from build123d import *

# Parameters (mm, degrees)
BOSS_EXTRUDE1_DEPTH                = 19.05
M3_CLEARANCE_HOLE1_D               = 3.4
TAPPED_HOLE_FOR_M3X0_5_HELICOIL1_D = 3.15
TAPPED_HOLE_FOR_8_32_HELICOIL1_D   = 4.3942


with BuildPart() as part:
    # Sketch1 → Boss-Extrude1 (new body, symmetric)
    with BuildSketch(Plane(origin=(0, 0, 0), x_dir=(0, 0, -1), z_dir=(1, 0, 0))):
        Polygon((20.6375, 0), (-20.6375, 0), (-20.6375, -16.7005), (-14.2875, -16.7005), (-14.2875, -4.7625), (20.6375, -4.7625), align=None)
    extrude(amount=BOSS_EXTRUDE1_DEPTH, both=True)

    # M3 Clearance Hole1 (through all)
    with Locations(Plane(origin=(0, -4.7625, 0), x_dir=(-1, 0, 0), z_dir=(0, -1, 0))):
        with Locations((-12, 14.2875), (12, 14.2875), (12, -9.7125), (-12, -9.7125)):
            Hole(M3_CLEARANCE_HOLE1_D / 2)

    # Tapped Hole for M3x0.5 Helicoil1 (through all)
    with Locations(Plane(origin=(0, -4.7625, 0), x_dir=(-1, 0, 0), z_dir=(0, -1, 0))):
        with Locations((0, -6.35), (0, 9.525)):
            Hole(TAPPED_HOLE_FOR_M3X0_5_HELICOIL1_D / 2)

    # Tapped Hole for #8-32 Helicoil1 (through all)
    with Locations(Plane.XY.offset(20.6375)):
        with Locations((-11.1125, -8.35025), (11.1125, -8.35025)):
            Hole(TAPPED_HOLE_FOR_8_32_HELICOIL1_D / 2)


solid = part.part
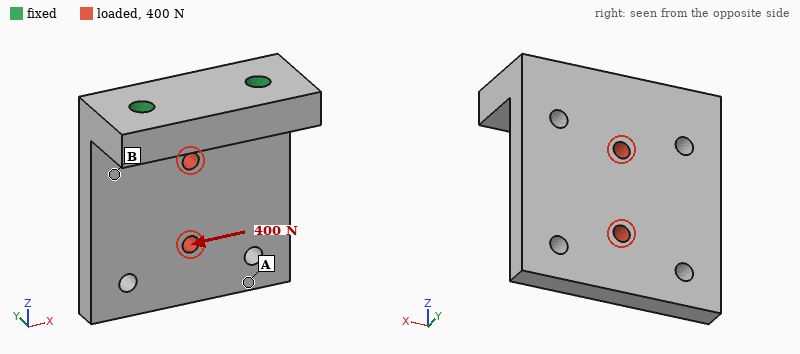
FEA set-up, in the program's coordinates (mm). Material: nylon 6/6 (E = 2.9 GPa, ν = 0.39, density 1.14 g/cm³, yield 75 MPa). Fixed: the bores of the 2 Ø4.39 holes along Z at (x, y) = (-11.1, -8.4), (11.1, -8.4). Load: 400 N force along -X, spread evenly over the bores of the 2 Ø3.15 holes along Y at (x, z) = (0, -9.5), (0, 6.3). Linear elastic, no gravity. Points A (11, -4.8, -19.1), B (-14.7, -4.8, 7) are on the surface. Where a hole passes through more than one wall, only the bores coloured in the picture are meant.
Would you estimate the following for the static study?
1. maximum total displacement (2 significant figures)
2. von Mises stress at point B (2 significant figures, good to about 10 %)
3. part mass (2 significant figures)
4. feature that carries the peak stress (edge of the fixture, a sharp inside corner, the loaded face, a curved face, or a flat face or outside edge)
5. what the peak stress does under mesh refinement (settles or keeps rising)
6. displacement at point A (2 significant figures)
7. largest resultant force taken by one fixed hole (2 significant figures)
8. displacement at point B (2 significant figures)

0.22 mm
6.0 MPa
11 g
edge of the fixture
keeps rising
0.20 mm
360 N
0.085 mm
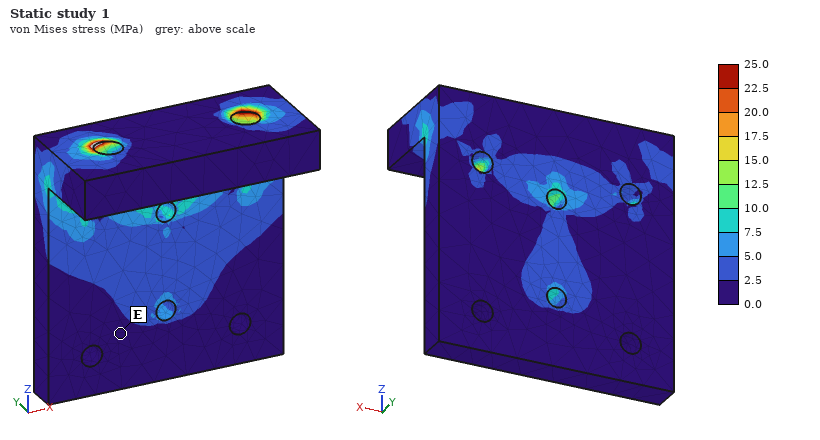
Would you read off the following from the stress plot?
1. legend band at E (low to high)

0.0 to 2.5 MPa
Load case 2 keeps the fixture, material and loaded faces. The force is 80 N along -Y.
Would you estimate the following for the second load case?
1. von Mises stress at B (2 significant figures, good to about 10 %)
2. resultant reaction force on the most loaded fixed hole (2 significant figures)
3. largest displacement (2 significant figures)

5.7 MPa
42 N
0.61 mm
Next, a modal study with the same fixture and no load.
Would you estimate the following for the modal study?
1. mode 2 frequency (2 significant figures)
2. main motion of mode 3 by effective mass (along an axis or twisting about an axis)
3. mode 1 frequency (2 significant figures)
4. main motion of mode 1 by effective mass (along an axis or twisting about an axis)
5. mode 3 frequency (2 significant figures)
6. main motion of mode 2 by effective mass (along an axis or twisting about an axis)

1900 Hz
along X
810 Hz
along Y
3000 Hz
twisting about Z
